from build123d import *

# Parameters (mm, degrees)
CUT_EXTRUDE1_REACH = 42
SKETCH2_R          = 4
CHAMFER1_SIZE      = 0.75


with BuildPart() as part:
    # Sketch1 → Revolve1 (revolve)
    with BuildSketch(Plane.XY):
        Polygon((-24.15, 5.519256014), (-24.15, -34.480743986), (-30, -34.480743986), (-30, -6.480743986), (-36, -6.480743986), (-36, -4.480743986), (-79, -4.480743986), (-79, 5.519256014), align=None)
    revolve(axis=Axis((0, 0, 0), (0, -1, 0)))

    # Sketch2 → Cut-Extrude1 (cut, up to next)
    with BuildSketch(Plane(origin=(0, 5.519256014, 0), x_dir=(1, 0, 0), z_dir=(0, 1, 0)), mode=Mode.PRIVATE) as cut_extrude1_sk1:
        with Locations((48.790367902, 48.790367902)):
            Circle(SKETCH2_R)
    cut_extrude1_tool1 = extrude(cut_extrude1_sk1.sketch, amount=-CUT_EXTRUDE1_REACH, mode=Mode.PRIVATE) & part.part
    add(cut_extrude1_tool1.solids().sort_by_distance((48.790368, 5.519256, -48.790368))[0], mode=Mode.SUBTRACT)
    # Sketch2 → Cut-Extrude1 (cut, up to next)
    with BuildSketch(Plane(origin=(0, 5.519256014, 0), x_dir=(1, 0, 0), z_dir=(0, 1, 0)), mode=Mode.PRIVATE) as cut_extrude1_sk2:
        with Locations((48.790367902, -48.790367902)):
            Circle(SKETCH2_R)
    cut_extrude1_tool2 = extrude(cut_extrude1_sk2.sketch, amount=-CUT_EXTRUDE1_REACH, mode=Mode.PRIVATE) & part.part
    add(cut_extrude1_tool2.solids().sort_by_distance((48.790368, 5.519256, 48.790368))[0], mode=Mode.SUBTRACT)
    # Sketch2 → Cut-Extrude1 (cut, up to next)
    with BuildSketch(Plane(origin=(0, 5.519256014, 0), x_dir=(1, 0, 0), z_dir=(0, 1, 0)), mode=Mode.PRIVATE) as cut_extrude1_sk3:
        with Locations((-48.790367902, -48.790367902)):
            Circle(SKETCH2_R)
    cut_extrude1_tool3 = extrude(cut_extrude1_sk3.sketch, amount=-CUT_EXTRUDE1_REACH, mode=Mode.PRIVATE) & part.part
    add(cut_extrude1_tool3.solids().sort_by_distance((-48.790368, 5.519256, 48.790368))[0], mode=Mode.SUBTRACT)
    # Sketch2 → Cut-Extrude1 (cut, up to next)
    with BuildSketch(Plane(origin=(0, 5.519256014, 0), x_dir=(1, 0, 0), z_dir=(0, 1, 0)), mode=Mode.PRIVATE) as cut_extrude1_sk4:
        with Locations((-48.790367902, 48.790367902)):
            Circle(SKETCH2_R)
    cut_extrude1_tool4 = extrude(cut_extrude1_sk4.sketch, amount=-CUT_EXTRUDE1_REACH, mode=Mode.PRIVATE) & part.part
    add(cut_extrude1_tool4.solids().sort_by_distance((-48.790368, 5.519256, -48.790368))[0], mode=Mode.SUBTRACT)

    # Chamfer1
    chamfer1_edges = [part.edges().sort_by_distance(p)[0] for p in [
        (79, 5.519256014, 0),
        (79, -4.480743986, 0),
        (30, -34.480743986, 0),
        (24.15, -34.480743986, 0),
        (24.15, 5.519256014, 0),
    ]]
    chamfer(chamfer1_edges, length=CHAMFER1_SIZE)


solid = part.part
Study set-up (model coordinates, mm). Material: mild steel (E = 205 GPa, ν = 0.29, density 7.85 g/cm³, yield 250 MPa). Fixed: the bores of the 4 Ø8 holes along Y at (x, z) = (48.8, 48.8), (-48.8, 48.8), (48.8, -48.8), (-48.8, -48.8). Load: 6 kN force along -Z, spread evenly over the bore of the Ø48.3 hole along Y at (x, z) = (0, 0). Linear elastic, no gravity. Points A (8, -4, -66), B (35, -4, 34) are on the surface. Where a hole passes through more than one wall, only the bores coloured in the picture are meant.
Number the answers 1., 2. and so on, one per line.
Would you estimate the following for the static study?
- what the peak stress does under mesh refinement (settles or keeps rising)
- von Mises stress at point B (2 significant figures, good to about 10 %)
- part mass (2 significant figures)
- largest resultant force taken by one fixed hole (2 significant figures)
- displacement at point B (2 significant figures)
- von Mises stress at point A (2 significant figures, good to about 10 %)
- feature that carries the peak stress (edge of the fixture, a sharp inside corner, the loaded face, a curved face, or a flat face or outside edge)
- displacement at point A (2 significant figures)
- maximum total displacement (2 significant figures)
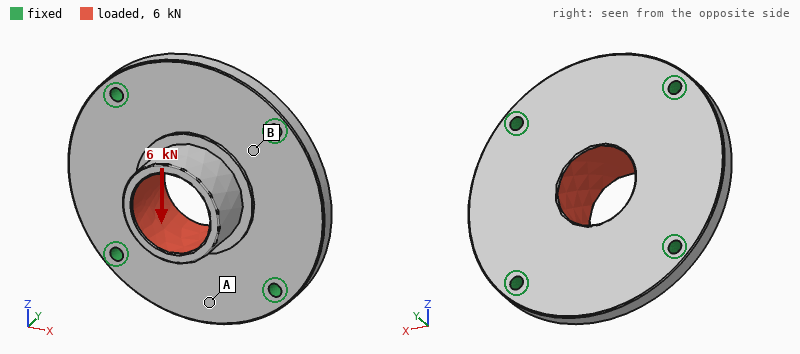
1. keeps rising
2. 8.0 MPa
3. 1.6 kg
4. 1.6 kN
5. 1.8 µm
6. 2.2 MPa
7. edge of the fixture
8. 3.1 µm
9. 9.4 µm
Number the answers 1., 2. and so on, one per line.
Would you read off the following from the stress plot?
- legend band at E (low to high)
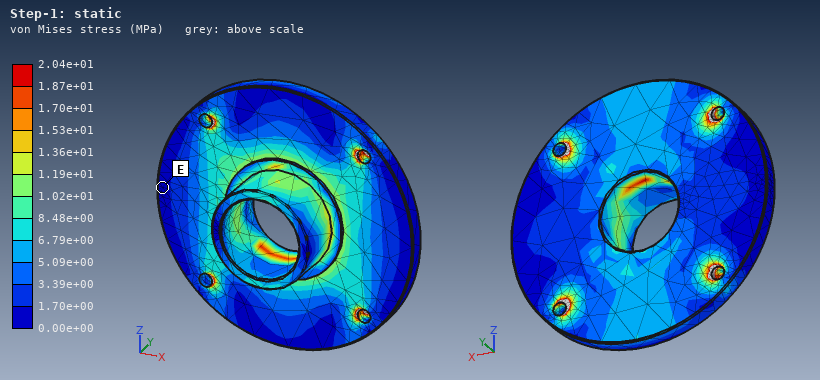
1. 0.00e+00 to 1.70e+00 MPa
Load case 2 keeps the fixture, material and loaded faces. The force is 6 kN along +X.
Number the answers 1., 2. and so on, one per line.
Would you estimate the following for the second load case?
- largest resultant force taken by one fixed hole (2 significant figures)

1. 1.6 kN
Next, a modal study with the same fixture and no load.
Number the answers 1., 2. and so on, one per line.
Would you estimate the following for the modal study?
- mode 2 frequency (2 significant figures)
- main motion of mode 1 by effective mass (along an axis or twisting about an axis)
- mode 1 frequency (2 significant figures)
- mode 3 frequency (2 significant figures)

1. 4400 Hz
2. along Y
3. 3800 Hz
4. 4400 Hz
